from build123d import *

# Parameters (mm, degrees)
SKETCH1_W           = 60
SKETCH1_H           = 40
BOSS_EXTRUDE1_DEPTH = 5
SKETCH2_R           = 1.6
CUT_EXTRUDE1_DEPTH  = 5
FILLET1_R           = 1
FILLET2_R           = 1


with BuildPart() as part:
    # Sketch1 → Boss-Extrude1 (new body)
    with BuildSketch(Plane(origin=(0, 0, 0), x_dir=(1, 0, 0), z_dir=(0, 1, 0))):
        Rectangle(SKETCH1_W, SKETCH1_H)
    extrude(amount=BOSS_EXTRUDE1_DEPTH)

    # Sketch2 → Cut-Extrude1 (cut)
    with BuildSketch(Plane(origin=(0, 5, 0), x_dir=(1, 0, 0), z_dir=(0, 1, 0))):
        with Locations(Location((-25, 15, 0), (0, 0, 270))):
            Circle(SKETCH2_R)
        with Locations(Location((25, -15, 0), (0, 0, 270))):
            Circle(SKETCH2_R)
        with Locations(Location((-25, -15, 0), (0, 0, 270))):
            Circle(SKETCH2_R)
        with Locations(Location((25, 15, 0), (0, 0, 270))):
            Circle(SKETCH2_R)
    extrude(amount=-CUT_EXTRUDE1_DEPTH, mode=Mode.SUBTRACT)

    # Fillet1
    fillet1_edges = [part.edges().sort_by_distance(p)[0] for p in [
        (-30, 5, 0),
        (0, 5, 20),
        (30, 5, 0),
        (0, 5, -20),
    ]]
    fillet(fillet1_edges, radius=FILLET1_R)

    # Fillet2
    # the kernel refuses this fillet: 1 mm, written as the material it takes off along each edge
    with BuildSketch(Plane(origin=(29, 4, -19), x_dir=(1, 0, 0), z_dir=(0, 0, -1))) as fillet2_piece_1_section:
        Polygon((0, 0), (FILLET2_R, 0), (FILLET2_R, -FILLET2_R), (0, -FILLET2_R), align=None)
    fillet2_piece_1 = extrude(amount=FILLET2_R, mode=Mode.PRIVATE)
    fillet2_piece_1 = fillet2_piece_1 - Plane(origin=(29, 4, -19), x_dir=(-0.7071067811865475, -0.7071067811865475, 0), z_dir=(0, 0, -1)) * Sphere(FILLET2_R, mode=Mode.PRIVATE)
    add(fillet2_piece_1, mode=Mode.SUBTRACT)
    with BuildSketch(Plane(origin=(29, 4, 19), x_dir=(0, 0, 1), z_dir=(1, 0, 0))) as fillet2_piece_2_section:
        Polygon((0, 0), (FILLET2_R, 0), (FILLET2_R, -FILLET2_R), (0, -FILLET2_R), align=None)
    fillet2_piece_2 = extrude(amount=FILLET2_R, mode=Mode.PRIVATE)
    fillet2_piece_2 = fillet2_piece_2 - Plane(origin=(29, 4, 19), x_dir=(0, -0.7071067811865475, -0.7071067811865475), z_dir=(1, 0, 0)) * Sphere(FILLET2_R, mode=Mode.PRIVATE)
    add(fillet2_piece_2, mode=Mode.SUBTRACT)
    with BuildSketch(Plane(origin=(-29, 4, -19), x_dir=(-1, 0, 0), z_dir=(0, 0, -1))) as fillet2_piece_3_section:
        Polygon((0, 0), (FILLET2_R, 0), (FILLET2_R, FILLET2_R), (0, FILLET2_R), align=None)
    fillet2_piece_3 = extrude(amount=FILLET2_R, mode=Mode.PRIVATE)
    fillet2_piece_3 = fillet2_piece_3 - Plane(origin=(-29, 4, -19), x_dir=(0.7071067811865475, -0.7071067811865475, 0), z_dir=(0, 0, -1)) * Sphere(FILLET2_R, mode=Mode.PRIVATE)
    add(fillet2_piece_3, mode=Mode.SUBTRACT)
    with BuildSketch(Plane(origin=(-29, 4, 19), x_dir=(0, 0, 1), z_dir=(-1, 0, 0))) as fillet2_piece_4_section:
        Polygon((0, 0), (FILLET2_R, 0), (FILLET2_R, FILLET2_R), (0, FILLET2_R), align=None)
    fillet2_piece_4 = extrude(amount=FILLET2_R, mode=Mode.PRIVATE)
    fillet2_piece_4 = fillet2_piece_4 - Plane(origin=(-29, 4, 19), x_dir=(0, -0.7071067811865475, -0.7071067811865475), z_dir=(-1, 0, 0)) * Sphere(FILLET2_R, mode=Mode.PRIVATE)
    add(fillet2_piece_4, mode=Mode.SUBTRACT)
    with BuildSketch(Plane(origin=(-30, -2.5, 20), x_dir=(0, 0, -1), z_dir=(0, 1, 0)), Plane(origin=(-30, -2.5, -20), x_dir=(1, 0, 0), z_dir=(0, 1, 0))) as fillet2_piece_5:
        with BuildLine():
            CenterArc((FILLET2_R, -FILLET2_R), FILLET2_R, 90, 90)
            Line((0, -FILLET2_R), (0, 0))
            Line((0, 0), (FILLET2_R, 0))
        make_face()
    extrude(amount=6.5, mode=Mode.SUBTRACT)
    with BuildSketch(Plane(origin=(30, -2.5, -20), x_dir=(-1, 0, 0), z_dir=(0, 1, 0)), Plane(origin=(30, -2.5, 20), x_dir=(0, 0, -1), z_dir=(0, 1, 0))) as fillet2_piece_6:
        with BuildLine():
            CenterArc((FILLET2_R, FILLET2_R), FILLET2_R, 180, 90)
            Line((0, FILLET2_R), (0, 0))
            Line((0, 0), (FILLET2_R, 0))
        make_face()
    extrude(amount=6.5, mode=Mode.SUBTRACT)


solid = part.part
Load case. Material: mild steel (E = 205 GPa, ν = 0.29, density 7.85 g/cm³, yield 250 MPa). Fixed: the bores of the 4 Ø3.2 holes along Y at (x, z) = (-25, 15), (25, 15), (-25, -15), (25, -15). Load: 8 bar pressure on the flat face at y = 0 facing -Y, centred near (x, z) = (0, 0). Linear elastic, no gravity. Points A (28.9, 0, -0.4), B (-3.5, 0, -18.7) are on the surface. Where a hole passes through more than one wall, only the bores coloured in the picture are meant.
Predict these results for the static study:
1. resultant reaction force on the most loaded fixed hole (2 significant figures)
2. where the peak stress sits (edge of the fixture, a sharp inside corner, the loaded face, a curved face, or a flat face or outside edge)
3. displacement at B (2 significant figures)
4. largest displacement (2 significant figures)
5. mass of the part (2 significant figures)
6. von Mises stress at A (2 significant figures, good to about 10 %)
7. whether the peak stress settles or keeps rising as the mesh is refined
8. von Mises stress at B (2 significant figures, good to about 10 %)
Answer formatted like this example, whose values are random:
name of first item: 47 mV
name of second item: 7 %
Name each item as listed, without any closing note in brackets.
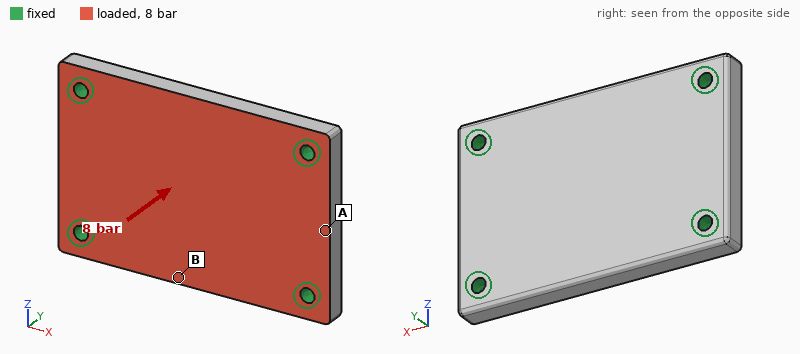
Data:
resultant reaction force on the most loaded fixed hole: 470 N
where the peak stress sits: edge of the fixture
displacement at B: 8.2 µm
largest displacement: 9.1 µm
mass of the part: 93 g
von Mises stress at A: 7.7 MPa
whether the peak stress settles or keeps rising as the mesh is refined: keeps rising
von Mises stress at B: 23 MPa
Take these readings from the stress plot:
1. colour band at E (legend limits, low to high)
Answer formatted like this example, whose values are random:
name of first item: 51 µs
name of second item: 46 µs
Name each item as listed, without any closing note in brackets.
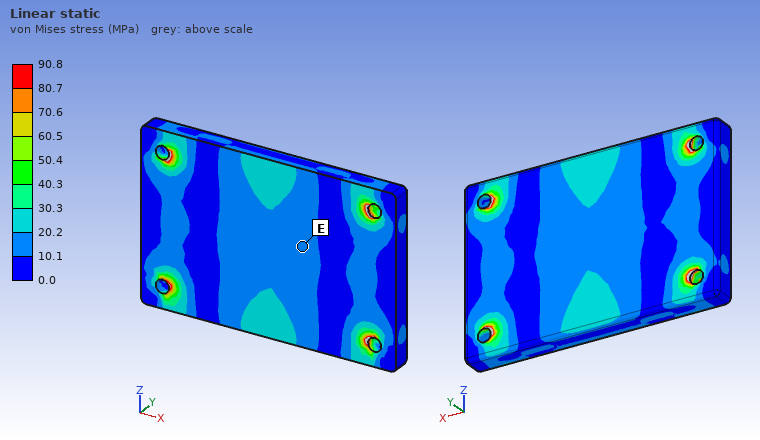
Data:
colour band at E: 10.1 to 20.2 MPa
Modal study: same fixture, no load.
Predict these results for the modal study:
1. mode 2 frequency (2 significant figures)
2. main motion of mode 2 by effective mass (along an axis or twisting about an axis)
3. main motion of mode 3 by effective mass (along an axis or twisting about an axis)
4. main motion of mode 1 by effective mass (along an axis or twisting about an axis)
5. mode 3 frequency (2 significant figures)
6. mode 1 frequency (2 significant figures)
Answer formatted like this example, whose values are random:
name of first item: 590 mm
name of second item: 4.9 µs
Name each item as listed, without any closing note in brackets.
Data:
mode 2 frequency: 13 kHz
main motion of mode 2 by effective mass: twisting about X
main motion of mode 3 by effective mass: twisting about Z
main motion of mode 1 by effective mass: along Y
mode 3 frequency: 21 kHz
mode 1 frequency: 8600 Hz
